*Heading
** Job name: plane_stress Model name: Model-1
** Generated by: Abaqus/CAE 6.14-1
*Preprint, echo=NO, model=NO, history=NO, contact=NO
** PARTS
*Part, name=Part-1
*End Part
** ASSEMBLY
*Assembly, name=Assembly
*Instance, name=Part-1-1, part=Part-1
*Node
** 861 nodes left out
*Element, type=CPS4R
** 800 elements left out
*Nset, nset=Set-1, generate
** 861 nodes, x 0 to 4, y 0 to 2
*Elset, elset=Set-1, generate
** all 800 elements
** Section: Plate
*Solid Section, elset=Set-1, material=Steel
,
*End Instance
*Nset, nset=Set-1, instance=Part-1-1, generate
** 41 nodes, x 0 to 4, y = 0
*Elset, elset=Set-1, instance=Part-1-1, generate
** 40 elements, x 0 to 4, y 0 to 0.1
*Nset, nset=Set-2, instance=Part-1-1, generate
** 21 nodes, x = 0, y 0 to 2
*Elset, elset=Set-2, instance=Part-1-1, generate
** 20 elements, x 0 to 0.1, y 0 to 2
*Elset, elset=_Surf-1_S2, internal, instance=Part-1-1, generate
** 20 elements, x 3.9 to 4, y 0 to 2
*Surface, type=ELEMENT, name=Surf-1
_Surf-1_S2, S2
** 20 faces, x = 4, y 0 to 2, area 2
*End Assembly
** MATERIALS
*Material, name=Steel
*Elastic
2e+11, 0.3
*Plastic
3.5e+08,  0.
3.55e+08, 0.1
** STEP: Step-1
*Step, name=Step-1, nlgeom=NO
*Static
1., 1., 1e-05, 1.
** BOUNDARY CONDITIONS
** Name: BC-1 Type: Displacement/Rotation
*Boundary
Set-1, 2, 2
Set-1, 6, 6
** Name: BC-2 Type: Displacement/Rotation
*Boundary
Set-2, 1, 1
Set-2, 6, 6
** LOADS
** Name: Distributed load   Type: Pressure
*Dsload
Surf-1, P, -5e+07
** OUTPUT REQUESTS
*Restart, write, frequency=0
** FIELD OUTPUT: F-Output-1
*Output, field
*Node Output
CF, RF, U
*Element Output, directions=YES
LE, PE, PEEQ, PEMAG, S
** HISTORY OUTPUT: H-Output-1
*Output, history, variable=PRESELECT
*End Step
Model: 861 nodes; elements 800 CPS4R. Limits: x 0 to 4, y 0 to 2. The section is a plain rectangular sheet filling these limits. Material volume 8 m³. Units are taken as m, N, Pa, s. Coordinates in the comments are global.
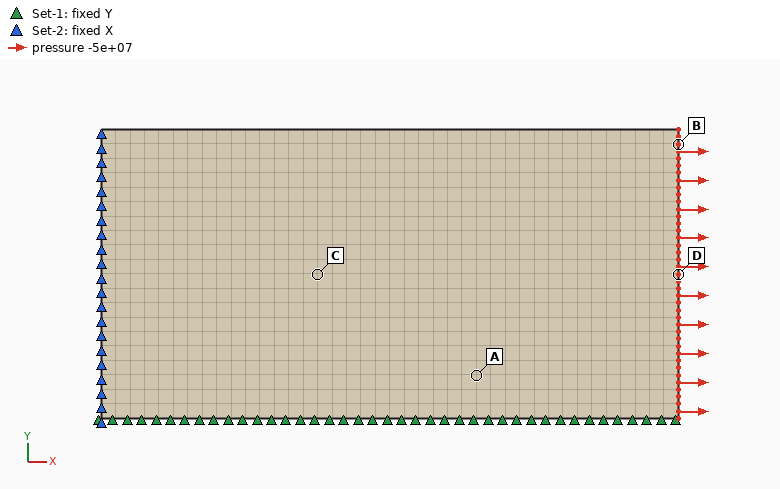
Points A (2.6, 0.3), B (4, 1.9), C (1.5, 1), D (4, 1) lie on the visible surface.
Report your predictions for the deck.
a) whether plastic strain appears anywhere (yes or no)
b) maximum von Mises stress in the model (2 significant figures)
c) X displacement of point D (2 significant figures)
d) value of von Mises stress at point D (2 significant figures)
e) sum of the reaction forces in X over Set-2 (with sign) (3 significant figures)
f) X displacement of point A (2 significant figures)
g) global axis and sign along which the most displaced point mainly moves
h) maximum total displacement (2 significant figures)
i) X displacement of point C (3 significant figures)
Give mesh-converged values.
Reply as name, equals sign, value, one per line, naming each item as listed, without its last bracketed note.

whether plastic strain appears anywhere = no
maximum von Mises stress in the model = 5.0e+07 Pa
X displacement of point D = 0.0010 m
value of von Mises stress at point D = 5.0e+07 Pa
sum of the reaction forces in X over Set-2 (with sign) = -1.00e+08 N
X displacement of point A = 6.5e-04 m
global axis and sign along which the most displaced point mainly moves = +X
maximum total displacement = 0.0010 m
X displacement of point C = 3.75e-04 m
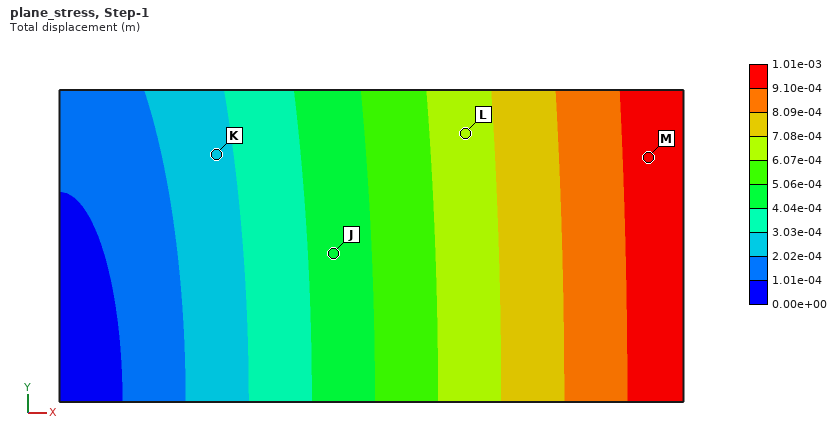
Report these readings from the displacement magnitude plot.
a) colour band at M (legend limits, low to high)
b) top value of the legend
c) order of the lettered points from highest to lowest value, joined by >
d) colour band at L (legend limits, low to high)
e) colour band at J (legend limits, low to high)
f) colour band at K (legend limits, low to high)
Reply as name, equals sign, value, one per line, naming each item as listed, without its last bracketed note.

colour band at M = 9.10e-04 to 1.01e-03 m
top value of the legend = 1.01e-03 m
order of the lettered points from highest to lowest value, joined by > = M > L > J > K
colour band at L = 6.07e-04 to 7.08e-04 m
colour band at J = 4.04e-04 to 5.06e-04 m
colour band at K = 2.02e-04 to 3.03e-04 m
